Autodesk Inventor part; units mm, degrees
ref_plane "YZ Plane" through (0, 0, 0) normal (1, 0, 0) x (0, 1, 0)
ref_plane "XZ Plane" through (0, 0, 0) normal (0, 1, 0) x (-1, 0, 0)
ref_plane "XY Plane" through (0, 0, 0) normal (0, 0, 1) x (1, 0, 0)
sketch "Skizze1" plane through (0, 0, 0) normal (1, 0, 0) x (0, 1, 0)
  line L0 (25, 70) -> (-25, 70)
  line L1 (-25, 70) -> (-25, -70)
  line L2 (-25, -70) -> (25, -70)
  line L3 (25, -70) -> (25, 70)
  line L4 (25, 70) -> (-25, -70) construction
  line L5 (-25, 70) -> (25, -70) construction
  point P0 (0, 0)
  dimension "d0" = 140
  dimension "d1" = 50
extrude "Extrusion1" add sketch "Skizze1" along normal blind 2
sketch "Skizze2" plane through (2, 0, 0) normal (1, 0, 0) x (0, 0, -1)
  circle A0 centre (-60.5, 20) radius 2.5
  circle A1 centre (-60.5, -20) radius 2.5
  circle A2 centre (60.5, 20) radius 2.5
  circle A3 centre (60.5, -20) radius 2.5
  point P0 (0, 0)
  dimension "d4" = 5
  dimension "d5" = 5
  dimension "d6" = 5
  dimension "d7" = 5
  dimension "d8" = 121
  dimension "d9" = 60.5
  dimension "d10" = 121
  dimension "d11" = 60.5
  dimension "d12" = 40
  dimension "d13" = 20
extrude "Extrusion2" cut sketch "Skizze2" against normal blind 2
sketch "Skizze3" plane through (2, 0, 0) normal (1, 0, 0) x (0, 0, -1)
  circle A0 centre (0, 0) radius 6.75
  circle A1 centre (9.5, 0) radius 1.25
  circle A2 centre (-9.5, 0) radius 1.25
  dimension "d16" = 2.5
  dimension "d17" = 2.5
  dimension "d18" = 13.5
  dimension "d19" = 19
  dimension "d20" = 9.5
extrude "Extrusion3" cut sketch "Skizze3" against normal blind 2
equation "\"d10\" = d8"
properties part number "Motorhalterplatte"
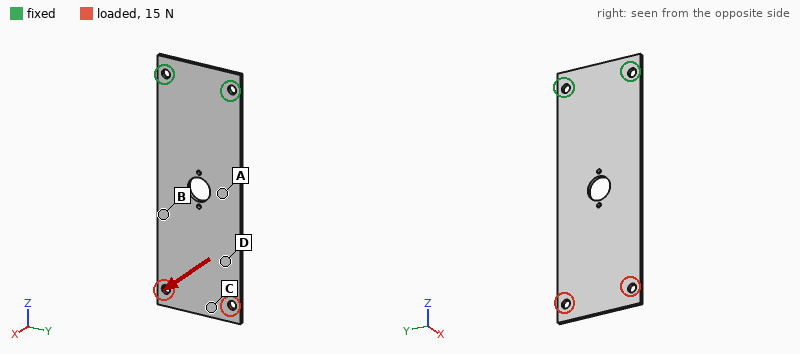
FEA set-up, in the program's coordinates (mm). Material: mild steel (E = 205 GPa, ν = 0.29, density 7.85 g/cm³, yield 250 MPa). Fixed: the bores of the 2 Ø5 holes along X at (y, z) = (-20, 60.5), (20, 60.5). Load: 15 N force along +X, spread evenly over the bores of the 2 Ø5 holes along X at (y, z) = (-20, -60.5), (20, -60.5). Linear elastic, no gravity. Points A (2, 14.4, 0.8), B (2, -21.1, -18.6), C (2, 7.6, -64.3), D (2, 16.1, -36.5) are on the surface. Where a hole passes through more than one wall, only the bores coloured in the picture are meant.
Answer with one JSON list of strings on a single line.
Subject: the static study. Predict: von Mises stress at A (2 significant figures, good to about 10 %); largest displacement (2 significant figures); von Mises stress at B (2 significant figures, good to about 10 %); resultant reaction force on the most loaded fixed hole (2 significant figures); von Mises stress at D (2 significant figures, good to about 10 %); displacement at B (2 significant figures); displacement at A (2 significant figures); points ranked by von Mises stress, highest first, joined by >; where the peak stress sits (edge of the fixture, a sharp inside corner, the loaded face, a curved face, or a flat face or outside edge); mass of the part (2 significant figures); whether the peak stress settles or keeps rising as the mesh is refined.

["37 MPa", "1.5 mm", "20 MPa", "7.5 N", "11 MPa", "0.67 mm", "0.41 mm", "A > B > D > C", "edge of the fixture", "110 g", "keeps rising"]
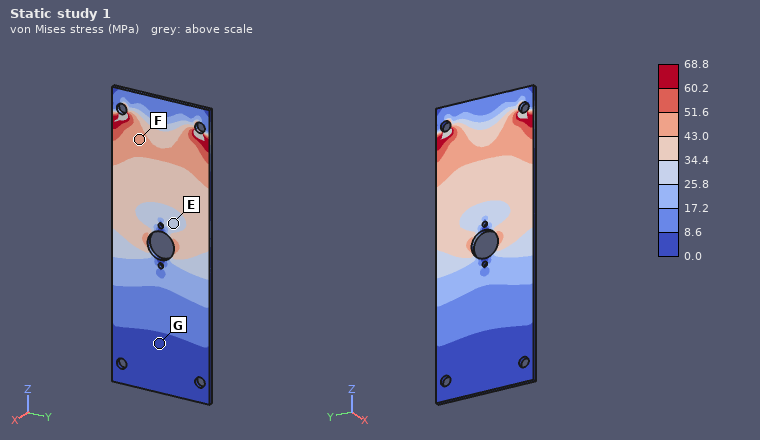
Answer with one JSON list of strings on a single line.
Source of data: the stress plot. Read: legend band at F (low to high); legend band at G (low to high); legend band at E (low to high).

["43.0 to 51.6 MPa", "0.0 to 8.6 MPa", "25.8 to 34.4 MPa"]
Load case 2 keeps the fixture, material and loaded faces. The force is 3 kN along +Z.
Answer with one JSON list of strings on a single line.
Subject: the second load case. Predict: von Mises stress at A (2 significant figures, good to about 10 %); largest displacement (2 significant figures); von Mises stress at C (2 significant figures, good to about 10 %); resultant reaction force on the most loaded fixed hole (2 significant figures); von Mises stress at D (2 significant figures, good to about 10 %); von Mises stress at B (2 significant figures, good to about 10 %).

["35 MPa", "25 µm", "16 MPa", "1.5 kN", "32 MPa", "35 MPa"]
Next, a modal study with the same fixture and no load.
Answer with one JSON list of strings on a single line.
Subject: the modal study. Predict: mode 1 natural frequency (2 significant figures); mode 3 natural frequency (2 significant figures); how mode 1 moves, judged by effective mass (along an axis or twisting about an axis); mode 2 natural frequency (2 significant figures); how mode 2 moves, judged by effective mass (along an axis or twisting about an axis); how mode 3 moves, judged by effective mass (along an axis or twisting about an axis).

["96 Hz", "600 Hz", "along X", "530 Hz", "twisting about Z", "along X"]
